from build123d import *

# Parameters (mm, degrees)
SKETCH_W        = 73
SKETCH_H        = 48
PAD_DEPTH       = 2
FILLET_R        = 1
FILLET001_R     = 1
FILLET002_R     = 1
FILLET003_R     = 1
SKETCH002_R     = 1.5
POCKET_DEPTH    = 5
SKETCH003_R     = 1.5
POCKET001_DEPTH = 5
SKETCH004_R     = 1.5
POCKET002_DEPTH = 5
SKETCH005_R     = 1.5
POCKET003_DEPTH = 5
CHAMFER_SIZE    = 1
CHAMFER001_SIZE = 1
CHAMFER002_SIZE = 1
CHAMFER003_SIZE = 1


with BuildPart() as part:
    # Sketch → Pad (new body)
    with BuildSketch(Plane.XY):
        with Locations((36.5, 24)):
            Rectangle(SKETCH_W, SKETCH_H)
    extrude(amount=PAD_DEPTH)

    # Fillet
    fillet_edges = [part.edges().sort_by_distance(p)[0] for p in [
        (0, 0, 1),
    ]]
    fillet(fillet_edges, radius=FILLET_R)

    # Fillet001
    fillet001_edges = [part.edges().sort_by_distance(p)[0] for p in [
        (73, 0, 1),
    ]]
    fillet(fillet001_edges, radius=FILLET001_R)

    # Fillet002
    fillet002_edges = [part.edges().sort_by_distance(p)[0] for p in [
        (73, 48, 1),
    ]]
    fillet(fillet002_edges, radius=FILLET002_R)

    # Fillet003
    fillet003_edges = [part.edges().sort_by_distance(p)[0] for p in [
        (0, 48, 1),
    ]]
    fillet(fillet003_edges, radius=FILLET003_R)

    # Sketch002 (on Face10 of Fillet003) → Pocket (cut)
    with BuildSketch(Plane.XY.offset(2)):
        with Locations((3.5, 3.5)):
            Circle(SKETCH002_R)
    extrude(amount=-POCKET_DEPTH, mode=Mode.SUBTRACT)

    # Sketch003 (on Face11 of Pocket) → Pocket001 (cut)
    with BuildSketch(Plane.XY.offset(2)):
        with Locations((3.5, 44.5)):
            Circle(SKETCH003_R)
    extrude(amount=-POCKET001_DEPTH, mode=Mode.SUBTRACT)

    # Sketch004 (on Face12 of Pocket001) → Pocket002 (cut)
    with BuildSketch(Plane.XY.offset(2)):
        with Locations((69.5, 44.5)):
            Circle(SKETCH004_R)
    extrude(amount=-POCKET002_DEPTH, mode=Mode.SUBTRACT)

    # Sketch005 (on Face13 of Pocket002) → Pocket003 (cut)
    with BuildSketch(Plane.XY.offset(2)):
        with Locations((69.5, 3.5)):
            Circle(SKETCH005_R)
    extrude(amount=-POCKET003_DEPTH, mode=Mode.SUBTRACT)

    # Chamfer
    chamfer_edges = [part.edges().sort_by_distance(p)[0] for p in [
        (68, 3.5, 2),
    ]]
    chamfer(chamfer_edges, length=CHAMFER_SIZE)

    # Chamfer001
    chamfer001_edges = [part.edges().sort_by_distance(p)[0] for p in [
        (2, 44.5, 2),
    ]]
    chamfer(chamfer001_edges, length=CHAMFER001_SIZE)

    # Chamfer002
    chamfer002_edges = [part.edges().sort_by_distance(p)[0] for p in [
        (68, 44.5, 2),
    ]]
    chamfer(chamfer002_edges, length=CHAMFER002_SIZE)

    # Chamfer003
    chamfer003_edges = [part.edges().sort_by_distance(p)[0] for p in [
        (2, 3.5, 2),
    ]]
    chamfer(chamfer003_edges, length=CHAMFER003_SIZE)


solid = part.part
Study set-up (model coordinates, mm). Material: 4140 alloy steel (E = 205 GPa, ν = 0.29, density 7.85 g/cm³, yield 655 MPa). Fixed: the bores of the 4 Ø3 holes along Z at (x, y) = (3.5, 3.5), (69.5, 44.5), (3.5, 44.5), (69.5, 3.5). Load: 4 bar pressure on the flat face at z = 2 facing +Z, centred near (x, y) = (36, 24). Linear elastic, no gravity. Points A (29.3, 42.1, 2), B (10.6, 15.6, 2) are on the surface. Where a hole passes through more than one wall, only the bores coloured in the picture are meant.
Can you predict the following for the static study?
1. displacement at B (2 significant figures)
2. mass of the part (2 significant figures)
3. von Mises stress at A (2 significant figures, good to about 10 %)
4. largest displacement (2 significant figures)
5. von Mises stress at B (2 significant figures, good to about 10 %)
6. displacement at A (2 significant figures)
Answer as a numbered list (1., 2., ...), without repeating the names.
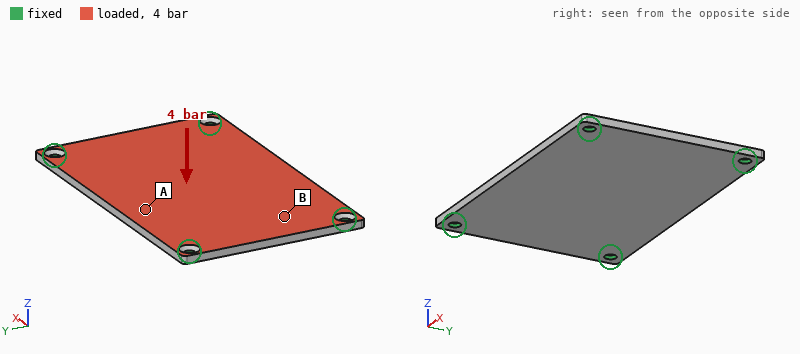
1. 0.090 mm
2. 54 g
3. 140 MPa
4. 0.26 mm
5. 67 MPa
6. 0.22 mm
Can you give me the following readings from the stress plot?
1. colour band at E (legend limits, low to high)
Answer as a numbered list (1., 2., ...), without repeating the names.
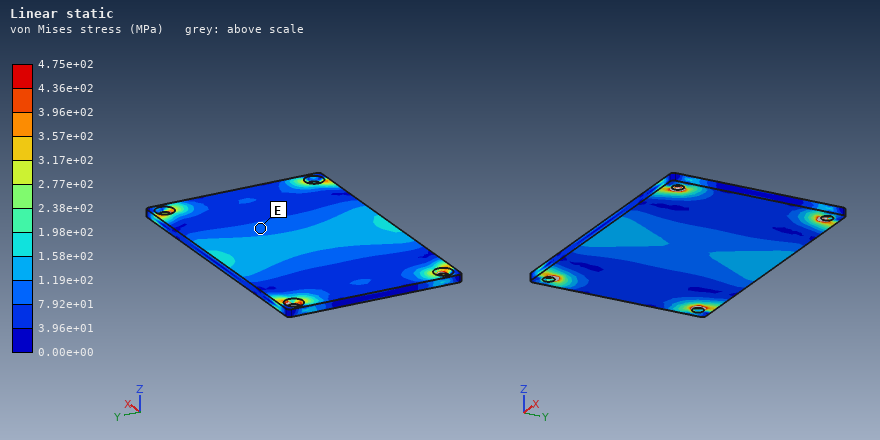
1. 7.92e+01 to 1.19e+02 MPa
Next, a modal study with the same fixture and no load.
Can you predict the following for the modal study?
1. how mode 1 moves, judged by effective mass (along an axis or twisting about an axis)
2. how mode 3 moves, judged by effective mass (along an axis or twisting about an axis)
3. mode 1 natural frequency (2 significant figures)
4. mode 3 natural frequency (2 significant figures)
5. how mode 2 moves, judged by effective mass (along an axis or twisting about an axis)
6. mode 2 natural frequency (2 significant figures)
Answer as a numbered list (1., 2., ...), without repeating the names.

1. along Z
2. twisting about Y
3. 1800 Hz
4. 4700 Hz
5. twisting about X
6. 3100 Hz
